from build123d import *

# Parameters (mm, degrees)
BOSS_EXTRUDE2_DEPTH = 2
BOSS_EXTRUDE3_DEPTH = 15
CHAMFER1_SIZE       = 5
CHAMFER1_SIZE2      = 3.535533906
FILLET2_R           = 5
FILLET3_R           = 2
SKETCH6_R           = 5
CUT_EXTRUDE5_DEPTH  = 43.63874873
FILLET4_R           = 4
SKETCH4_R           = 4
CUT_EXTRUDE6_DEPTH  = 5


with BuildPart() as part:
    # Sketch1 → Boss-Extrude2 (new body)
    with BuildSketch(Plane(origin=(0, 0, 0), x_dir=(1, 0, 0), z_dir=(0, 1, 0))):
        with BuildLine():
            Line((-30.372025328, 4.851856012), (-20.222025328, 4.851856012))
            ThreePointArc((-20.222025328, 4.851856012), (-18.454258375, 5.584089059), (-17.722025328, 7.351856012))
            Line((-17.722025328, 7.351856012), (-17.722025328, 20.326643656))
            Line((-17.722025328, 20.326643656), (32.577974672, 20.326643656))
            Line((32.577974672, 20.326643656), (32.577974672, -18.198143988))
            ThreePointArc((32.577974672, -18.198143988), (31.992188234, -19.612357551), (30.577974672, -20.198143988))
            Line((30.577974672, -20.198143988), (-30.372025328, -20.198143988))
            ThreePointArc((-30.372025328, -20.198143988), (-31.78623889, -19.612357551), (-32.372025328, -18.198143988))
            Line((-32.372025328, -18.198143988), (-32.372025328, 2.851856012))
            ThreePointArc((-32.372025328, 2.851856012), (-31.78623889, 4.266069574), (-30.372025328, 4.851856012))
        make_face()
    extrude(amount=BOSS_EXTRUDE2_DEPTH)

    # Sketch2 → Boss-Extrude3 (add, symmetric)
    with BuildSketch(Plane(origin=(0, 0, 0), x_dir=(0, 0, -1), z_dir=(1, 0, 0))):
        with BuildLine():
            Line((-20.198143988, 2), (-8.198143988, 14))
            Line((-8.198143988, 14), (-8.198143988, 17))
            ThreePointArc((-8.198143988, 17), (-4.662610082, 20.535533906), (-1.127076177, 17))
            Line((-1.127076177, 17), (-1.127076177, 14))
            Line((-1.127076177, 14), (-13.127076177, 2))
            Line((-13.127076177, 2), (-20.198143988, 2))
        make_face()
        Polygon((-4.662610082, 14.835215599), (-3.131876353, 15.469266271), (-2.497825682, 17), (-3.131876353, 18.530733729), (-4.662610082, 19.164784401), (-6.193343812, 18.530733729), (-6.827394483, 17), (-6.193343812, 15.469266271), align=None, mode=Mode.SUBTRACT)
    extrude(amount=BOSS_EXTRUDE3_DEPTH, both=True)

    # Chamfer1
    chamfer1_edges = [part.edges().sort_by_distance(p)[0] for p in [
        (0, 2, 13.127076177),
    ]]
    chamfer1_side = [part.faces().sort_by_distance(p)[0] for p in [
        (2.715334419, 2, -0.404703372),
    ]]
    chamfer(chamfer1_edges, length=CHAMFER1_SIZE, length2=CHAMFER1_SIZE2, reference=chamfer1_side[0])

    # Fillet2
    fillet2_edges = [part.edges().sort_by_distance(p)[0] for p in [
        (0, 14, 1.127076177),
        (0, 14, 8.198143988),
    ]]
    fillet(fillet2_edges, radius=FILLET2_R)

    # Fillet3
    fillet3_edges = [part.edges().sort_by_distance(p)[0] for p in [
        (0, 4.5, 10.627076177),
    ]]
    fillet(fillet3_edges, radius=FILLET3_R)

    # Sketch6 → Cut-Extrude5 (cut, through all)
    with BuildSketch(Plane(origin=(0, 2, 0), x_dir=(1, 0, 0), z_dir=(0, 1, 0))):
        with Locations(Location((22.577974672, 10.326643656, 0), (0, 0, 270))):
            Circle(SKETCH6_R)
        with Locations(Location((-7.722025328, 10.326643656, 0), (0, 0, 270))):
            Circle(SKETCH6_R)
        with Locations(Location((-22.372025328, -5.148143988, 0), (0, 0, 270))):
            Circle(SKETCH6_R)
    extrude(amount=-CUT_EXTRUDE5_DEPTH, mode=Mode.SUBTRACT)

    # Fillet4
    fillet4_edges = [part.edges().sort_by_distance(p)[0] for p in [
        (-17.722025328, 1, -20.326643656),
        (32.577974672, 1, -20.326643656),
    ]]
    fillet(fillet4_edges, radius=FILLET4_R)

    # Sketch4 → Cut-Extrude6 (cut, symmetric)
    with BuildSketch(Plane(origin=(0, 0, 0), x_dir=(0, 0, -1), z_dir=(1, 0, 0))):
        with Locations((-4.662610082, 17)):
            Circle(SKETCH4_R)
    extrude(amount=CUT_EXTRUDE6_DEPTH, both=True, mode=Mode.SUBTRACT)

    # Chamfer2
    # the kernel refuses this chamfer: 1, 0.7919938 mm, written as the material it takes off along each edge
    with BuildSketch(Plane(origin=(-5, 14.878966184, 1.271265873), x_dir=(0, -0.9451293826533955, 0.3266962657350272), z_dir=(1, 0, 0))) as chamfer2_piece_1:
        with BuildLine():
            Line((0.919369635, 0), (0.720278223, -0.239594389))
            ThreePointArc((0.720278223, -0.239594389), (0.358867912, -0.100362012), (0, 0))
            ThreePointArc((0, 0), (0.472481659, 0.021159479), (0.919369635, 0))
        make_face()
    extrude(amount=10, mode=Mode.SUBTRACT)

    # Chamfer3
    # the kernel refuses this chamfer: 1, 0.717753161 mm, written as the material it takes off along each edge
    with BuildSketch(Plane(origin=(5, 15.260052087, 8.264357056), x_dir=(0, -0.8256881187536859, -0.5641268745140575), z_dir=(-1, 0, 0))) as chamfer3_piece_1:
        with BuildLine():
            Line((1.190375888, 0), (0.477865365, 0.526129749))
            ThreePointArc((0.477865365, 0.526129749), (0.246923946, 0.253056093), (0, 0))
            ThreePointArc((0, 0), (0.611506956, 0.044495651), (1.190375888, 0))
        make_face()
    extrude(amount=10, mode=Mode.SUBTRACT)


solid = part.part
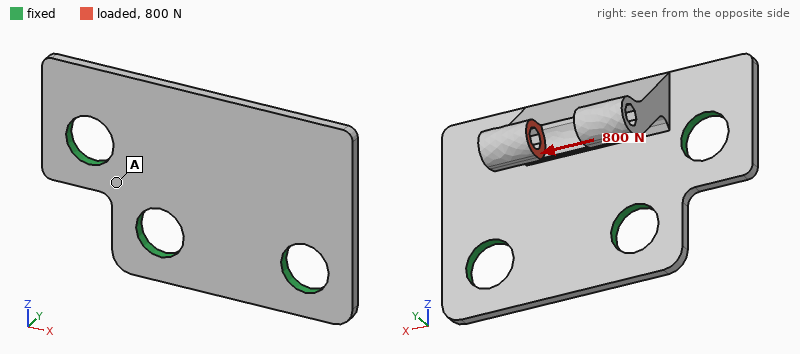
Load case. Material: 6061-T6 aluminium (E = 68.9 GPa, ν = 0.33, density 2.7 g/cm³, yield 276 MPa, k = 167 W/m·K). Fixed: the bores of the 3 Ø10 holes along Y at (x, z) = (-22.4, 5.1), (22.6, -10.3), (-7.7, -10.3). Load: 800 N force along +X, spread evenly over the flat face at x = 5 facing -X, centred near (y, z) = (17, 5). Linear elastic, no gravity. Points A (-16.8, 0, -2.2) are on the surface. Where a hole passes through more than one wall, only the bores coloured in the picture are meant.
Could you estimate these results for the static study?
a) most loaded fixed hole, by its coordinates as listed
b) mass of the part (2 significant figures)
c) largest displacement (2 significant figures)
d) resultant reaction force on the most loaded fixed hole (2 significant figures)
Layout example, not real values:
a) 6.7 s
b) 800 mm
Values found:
a) (-22.4, 5.1)
b) 21 g
c) 0.38 mm
d) 610 N
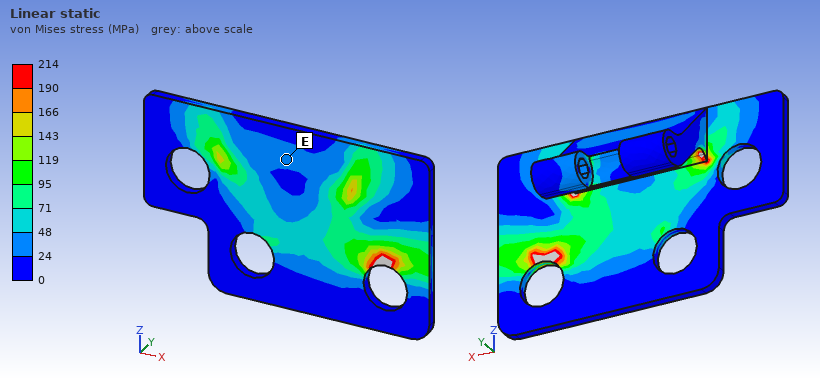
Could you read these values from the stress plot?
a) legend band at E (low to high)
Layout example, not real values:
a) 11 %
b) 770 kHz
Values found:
a) 24 to 48 MPa
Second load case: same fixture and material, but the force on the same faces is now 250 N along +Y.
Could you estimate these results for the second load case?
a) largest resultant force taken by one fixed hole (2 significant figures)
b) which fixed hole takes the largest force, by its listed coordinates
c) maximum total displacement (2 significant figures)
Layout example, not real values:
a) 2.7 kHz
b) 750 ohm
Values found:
a) 120 N
b) (22.6, -10.3)
c) 94 µm
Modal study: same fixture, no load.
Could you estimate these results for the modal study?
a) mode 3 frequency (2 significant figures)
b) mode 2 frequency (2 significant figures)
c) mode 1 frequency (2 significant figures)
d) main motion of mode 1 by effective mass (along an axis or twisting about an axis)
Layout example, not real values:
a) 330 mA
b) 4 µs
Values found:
a) 7100 Hz
b) 4500 Hz
c) 2100 Hz
d) along Y
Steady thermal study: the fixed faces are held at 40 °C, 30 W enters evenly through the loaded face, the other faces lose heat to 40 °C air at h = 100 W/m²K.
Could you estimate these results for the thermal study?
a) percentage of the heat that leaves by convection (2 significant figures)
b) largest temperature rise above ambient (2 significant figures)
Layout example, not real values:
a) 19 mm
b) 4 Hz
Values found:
a) 28 %
b) 76 K
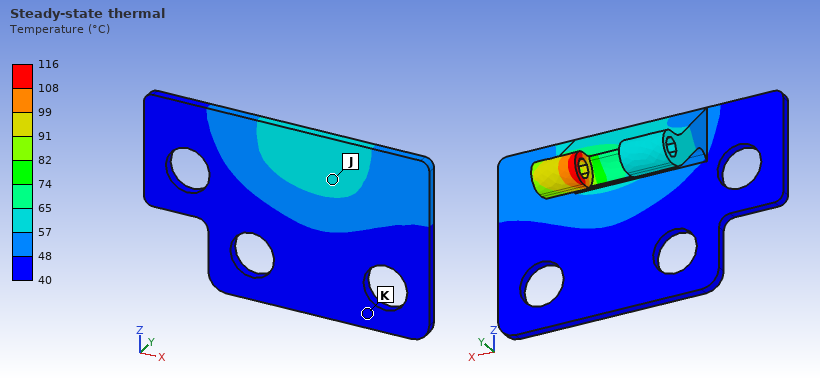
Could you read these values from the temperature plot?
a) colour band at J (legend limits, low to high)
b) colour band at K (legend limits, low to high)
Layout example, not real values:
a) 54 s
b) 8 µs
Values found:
a) 57 to 65 °C
b) 40 to 48 °C
